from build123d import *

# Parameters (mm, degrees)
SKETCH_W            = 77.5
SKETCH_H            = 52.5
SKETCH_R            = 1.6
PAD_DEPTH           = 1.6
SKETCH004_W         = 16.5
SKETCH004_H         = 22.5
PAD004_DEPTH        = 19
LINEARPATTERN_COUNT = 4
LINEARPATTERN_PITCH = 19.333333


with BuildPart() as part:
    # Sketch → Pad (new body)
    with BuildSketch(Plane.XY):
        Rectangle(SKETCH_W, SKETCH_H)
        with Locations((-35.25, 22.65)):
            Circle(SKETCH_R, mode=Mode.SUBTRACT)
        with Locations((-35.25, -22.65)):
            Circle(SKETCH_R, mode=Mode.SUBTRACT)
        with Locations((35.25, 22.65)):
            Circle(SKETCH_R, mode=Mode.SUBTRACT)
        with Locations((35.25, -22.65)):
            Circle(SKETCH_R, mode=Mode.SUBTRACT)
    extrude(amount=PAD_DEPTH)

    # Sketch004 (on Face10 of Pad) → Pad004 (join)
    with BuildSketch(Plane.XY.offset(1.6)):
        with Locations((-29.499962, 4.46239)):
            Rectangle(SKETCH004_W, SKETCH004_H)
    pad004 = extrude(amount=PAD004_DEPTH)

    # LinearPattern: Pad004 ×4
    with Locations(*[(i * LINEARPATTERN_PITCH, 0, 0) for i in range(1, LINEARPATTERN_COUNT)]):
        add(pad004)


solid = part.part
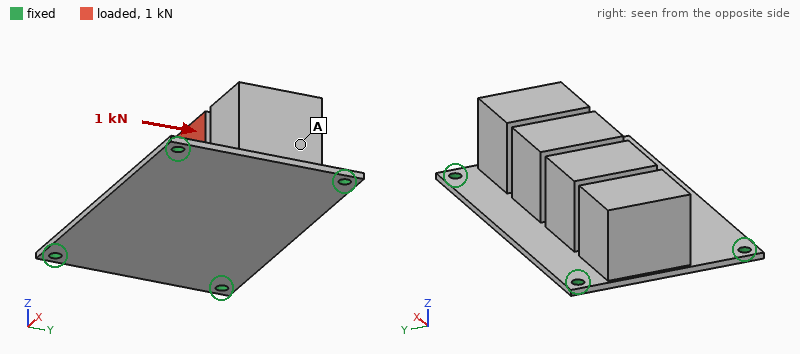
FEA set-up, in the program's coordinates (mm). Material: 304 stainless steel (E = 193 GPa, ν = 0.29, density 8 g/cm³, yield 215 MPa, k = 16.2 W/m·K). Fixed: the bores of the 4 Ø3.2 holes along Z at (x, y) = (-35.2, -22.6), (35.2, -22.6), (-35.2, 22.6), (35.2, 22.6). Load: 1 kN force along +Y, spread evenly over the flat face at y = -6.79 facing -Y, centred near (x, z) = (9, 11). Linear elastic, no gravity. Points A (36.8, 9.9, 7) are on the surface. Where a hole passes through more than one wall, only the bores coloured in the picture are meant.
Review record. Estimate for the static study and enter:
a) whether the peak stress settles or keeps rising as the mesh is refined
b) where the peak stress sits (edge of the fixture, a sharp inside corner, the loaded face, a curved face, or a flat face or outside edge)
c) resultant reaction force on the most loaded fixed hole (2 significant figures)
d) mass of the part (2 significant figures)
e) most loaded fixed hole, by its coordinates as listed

keeps rising
edge of the fixture
410 N
280 g
(35.2, 22.6)
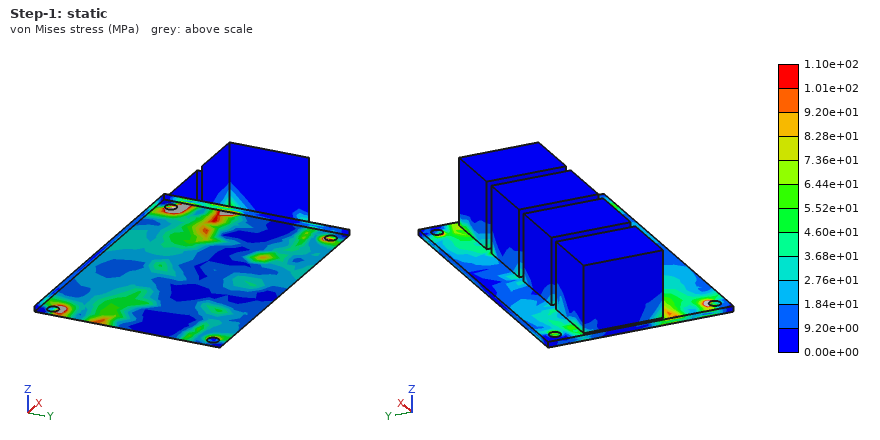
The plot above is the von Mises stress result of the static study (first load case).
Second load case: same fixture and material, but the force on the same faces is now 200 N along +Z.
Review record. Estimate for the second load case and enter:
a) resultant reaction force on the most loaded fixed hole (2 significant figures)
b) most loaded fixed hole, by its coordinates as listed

89 N
(35.2, -22.6)
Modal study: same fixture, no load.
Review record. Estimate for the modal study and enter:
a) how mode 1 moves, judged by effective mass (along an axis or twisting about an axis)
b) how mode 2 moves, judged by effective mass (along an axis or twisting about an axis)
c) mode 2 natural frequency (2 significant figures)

along Z
along Y
1700 Hz
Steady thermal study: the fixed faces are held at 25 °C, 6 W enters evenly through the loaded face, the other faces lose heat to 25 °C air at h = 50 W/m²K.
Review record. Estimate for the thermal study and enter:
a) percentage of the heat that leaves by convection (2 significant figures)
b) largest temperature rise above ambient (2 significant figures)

90 %
34 K
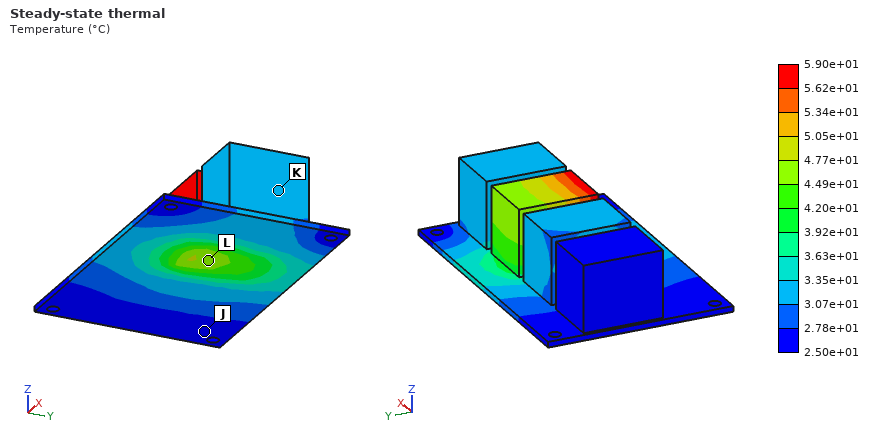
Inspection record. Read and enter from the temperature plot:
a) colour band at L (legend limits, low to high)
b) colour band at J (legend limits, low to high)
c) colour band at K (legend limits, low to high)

4.49e+01 to 4.77e+01 °C
2.50e+01 to 2.78e+01 °C
3.07e+01 to 3.35e+01 °C
